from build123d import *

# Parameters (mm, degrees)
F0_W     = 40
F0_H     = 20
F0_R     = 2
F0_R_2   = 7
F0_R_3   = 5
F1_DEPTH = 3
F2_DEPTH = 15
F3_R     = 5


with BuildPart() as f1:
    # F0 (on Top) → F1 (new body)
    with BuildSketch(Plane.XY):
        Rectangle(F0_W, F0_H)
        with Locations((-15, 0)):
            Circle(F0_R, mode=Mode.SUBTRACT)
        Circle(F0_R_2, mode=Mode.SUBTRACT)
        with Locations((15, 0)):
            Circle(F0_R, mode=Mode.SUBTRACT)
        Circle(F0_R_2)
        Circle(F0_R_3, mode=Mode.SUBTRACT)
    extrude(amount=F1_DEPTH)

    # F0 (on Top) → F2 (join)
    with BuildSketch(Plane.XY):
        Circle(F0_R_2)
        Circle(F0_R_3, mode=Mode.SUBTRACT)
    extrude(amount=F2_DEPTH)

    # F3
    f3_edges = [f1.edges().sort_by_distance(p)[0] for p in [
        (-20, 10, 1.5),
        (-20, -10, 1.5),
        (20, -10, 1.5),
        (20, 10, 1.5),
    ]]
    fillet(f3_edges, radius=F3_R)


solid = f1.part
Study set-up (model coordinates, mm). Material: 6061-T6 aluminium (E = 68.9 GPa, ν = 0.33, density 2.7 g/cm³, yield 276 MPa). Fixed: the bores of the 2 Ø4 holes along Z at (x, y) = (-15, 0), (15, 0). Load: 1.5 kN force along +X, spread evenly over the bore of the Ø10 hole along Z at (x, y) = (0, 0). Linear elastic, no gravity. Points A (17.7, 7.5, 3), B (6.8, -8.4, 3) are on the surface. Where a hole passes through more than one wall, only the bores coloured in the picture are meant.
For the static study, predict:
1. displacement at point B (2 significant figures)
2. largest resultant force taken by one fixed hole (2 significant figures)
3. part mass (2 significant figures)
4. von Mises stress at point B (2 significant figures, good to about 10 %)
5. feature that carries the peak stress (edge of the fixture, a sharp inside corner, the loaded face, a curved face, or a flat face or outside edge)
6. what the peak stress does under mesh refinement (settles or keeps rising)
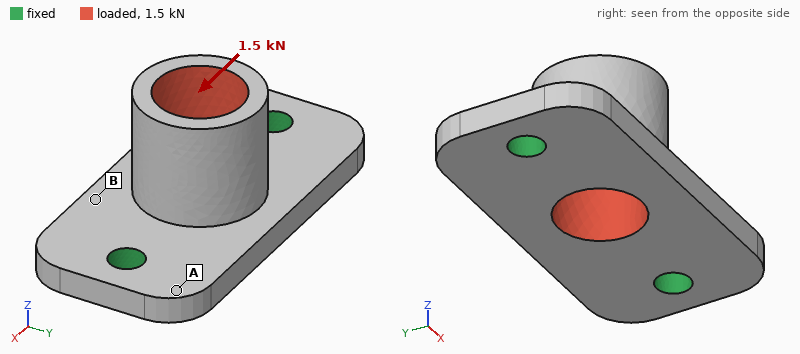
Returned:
8.3 µm
860 N
7.9 g
35 MPa
edge of the fixture
keeps rising
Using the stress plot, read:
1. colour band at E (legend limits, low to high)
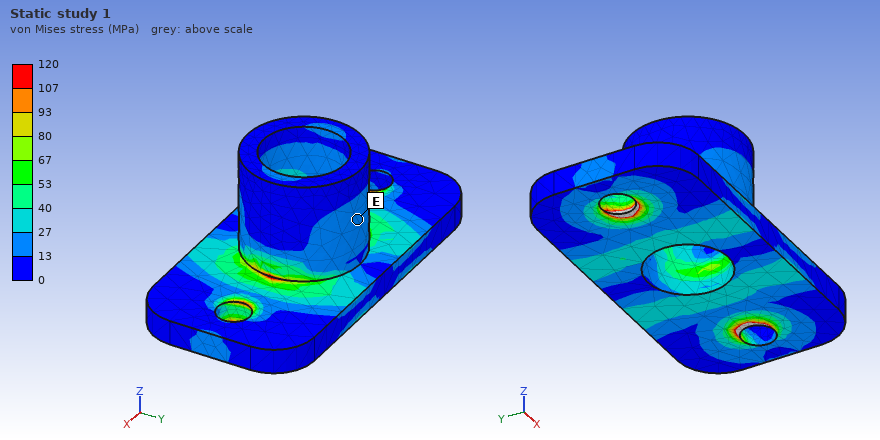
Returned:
13 to 27 MPa
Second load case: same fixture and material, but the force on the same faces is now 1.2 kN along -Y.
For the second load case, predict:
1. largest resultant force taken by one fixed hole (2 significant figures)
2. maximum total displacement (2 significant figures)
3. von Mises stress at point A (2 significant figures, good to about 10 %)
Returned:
600 N
0.12 mm
33 MPa
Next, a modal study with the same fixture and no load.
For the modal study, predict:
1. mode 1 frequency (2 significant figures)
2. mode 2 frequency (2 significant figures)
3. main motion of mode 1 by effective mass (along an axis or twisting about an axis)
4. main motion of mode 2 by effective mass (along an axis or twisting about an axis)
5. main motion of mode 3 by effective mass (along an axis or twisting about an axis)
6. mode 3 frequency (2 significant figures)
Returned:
8900 Hz
15 kHz
along Y
along Z
along X
19 kHz
